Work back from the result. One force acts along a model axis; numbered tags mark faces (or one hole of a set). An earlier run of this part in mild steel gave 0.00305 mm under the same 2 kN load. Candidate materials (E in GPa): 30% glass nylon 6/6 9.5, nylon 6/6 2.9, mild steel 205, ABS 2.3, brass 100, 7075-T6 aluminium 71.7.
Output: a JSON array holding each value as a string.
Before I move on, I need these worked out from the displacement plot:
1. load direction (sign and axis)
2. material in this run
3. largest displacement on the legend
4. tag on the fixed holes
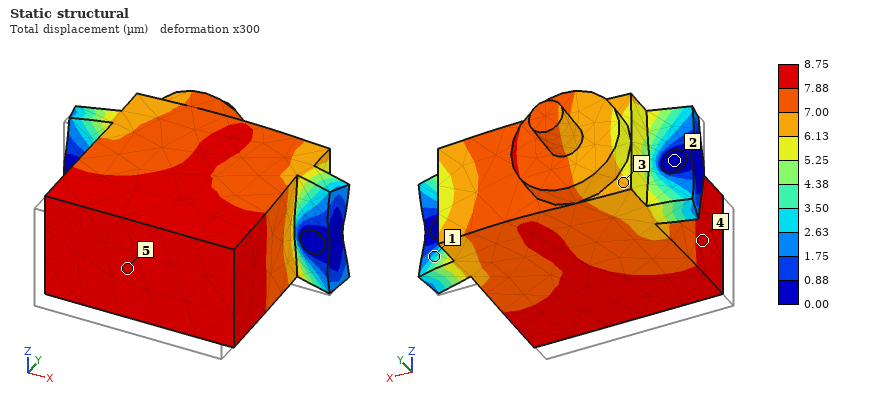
["+Y", "7075-T6 aluminium", "8.75 µm", "2"]
